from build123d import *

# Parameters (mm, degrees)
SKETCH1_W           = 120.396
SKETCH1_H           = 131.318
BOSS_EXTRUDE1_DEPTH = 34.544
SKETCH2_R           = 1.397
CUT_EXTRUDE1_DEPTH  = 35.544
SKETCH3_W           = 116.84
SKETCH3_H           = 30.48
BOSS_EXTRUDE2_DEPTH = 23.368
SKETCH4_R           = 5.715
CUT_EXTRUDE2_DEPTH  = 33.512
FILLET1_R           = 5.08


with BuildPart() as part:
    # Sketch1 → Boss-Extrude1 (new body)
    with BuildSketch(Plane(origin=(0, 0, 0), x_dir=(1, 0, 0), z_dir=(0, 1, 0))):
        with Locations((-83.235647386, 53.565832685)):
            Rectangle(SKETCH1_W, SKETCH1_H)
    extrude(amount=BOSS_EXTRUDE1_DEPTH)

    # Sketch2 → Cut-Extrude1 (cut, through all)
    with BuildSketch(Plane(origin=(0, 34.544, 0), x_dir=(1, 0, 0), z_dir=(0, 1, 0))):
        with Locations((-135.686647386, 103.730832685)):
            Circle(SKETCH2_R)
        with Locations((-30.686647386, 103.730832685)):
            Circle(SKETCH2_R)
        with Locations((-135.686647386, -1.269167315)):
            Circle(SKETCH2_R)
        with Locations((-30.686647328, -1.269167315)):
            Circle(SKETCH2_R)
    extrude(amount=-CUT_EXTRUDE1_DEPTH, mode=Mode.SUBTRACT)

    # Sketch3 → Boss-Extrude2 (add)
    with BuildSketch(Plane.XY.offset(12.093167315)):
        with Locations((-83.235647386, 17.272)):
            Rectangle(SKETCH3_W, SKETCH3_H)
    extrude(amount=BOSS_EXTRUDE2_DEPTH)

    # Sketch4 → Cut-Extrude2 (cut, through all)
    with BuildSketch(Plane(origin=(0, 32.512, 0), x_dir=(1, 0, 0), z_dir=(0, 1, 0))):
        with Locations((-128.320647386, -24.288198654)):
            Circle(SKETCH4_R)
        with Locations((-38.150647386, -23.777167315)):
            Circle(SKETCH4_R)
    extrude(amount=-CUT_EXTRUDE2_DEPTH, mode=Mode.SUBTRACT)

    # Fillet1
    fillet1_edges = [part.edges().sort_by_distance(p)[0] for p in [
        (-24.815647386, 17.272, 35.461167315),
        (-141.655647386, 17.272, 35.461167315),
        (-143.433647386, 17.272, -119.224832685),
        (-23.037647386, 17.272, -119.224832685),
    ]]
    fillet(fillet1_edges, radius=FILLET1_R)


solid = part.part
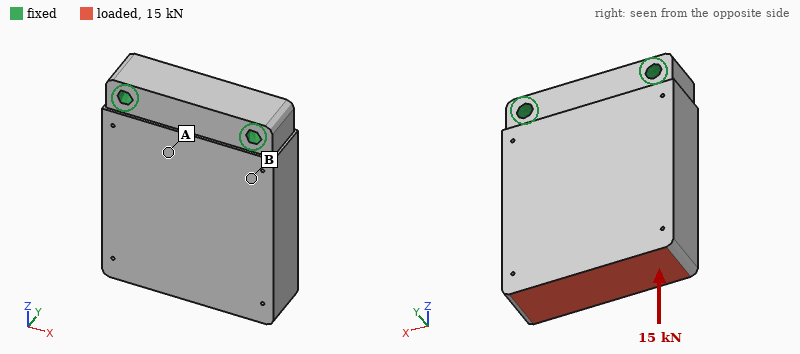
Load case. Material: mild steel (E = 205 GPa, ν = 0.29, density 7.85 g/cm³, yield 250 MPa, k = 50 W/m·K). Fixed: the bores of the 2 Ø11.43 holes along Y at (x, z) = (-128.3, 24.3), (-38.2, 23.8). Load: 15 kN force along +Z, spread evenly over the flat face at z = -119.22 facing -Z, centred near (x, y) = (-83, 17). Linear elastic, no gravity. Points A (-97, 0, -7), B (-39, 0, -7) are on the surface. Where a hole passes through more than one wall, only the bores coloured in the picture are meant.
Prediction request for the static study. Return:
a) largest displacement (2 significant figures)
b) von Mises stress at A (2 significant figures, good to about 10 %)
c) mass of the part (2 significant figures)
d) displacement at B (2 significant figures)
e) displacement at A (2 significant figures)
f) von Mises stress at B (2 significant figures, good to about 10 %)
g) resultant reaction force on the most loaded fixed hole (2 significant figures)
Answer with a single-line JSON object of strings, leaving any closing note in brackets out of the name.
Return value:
{"largest displacement": "3.2 µm", "von Mises stress at A": "2.4 MPa", "mass of the part": "4.9 kg", "displacement at B": "0.96 µm", "displacement at A": "1.3 µm", "von Mises stress at B": "5.1 MPa", "resultant reaction force on the most loaded fixed hole": "7.7 kN"}
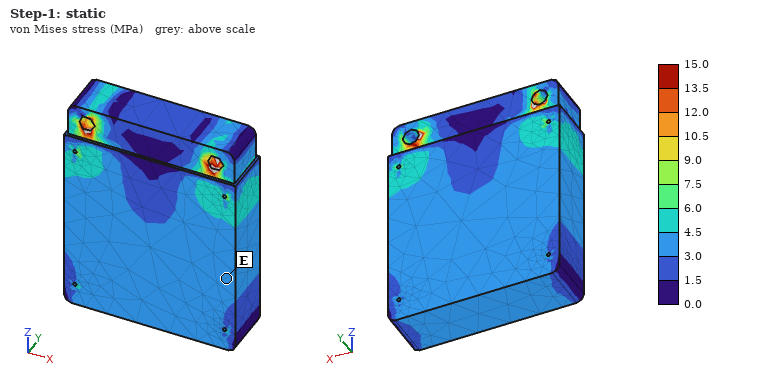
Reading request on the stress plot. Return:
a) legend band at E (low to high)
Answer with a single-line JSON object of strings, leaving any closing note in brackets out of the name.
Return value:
{"legend band at E": "3.0 to 4.5 MPa"}
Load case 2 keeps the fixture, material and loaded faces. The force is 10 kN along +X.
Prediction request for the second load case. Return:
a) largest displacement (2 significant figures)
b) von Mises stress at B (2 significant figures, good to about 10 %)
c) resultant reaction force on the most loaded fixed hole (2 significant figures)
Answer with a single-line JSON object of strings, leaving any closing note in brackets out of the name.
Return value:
{"largest displacement": "17 µm", "von Mises stress at B": "11 MPa", "resultant reaction force on the most loaded fixed hole": "16 kN"}
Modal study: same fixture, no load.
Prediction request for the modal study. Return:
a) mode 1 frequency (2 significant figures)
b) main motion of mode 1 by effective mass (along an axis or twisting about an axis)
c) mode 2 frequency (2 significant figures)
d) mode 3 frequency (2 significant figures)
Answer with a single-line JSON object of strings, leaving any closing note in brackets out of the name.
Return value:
{"mode 1 frequency": "1100 Hz", "main motion of mode 1 by effective mass": "along Y", "mode 2 frequency": "3100 Hz", "mode 3 frequency": "3200 Hz"}
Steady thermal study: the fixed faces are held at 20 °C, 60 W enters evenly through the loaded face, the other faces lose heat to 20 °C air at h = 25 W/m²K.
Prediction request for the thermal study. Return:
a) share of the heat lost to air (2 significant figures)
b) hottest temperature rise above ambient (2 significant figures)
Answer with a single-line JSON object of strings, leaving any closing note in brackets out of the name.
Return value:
{"share of the heat lost to air": "34 %", "hottest temperature rise above ambient": "36 K"}
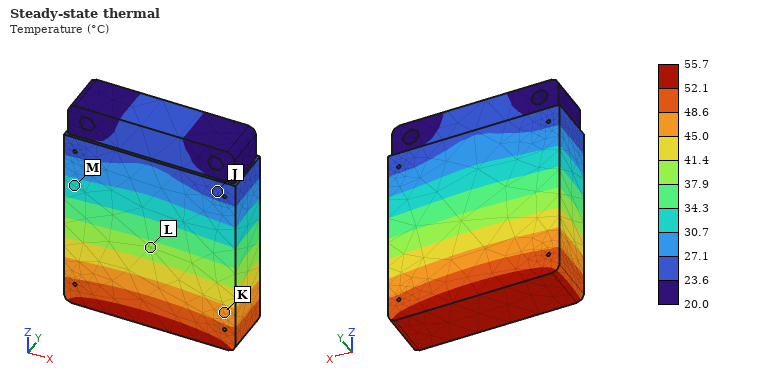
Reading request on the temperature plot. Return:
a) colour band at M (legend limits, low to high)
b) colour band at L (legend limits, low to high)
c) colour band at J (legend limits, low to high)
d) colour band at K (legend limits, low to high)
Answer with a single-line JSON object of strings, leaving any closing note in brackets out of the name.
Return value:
{"colour band at M": "30.7 to 34.3 °C", "colour band at L": "37.9 to 41.4 °C", "colour band at J": "23.6 to 27.1 °C", "colour band at K": "45.0 to 48.6 °C"}
